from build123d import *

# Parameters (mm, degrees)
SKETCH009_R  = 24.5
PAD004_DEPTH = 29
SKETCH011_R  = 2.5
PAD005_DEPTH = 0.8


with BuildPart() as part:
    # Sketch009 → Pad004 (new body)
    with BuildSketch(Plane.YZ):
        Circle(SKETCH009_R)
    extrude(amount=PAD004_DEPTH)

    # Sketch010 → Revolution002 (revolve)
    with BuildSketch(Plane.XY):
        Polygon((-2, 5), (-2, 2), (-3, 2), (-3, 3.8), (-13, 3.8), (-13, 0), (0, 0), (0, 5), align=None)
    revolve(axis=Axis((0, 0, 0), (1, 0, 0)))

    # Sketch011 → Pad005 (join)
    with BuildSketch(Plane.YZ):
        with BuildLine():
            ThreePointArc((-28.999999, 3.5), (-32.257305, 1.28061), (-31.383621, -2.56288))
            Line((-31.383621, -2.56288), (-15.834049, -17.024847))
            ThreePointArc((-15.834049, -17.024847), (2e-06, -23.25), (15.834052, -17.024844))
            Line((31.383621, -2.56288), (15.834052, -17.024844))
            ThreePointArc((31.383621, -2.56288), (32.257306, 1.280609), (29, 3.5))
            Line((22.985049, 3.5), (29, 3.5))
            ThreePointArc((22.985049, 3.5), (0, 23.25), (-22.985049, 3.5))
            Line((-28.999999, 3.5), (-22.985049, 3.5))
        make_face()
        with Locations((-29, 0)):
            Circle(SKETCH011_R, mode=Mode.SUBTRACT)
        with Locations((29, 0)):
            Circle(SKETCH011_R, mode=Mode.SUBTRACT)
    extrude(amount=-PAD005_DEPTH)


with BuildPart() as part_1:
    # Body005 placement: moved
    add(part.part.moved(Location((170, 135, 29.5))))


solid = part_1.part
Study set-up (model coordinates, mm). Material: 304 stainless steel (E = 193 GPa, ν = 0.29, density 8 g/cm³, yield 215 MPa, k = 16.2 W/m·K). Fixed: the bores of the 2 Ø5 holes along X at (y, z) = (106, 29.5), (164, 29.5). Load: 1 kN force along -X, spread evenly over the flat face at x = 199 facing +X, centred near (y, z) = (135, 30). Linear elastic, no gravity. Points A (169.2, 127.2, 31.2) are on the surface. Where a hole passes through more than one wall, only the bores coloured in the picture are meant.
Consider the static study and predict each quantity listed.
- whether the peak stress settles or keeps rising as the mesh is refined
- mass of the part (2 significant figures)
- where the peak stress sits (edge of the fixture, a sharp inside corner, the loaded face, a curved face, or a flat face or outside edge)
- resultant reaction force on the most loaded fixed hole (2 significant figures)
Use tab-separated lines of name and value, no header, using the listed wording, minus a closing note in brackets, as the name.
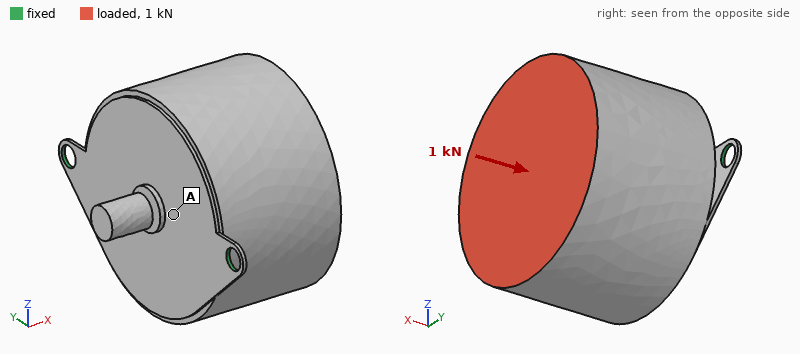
whether the peak stress settles or keeps rising as the mesh is refined	keeps rising
mass of the part	450 g
where the peak stress sits	edge of the fixture
resultant reaction force on the most loaded fixed hole	590 N
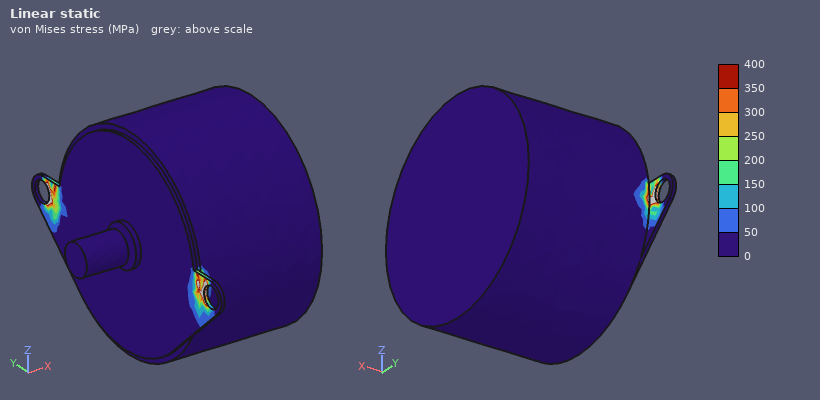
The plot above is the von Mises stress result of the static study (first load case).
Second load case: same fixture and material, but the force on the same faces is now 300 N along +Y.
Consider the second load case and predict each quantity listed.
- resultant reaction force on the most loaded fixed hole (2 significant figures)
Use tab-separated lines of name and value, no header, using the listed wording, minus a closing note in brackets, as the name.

resultant reaction force on the most loaded fixed hole	230 N
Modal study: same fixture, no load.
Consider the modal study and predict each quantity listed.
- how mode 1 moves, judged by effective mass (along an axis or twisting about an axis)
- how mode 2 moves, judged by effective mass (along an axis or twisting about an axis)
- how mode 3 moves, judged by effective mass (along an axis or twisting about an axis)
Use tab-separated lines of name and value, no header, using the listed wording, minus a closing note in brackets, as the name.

how mode 1 moves, judged by effective mass	along Z
how mode 2 moves, judged by effective mass	along X
how mode 3 moves, judged by effective mass	along Y
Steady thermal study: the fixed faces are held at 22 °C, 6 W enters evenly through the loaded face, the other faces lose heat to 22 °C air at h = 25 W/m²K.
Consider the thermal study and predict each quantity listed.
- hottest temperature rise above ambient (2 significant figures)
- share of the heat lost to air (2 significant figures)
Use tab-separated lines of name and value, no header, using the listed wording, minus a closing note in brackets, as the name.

hottest temperature rise above ambient	30 K
share of the heat lost to air	76 %
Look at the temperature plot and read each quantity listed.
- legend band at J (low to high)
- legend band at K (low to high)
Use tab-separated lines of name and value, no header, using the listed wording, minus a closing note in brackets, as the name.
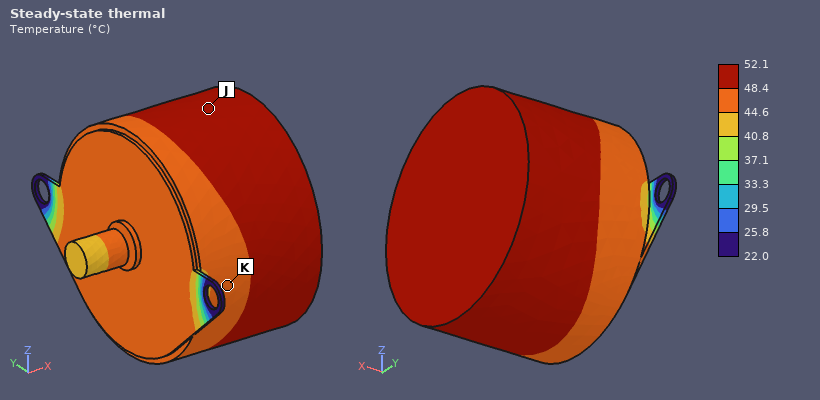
legend band at J	48.4 to 52.1 °C
legend band at K	44.6 to 48.4 °C
